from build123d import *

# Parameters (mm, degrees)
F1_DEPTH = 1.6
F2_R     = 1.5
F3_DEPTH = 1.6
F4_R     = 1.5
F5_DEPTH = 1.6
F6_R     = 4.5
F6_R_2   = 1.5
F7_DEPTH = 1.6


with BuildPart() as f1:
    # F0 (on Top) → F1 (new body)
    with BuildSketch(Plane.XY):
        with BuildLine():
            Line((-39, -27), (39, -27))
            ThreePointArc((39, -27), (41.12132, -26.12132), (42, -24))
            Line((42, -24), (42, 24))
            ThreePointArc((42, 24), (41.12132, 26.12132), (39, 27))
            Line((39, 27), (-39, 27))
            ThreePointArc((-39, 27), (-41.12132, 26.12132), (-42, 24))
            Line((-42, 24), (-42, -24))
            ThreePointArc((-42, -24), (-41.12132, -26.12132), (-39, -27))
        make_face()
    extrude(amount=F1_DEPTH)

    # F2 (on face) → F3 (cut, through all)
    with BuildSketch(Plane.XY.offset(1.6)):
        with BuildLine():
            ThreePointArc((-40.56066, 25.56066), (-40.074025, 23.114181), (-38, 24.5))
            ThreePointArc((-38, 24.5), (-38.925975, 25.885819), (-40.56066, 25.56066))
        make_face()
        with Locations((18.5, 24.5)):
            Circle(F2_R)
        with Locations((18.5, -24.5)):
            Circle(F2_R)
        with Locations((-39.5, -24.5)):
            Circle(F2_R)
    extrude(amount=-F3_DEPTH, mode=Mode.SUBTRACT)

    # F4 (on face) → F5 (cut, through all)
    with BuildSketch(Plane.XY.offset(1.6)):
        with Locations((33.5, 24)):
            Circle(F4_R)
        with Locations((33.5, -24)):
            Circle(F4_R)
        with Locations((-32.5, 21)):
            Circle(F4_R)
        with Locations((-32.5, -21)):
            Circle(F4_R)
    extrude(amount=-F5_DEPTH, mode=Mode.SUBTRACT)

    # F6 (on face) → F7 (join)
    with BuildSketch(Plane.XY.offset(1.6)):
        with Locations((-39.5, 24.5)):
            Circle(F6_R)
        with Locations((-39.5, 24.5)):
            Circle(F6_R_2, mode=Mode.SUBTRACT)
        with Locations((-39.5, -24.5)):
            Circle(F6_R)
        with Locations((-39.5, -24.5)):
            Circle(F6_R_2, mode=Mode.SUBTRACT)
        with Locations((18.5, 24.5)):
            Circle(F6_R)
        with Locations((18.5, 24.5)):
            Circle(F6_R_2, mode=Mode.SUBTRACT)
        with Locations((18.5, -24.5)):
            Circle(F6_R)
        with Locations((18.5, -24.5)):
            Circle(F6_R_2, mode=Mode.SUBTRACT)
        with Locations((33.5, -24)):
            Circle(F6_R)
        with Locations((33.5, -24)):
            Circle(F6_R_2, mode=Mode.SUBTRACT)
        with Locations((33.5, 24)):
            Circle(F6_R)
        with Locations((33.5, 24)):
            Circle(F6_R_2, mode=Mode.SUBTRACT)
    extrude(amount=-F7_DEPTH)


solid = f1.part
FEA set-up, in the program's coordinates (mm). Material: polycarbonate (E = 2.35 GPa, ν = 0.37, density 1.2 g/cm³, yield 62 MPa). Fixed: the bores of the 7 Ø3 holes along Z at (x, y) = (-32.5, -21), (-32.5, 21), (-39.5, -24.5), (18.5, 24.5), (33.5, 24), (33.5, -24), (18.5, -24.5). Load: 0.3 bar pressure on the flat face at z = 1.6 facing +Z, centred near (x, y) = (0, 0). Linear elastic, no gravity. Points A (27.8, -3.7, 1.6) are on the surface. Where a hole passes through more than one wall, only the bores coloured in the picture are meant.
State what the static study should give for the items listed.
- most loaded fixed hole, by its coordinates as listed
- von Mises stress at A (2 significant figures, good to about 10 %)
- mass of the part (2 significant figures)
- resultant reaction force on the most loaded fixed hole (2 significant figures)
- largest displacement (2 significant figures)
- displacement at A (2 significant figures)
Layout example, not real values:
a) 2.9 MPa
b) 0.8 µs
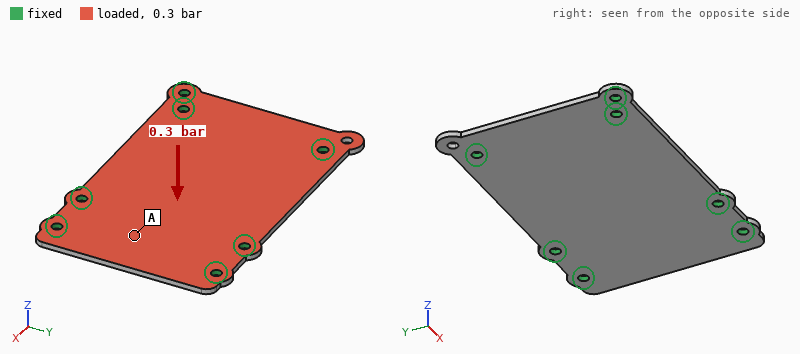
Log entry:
a) (-32.5, -21)
b) 6.6 MPa
c) 8.7 g
d) 33 N
e) 1.2 mm
f) 0.52 mm
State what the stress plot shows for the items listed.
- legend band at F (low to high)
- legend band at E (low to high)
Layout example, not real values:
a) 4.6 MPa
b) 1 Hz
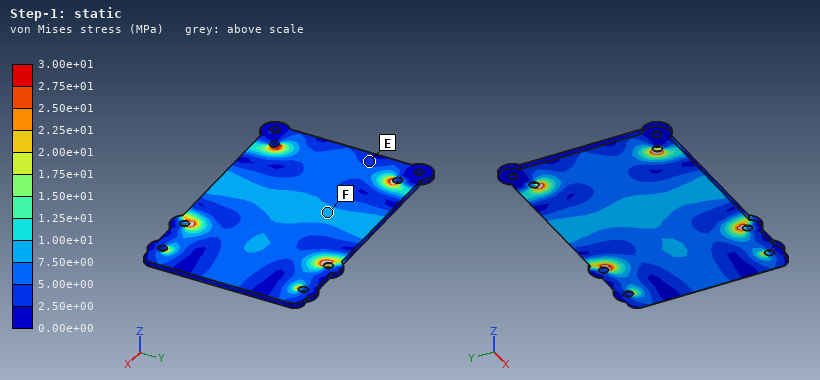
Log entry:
a) 7.50e+00 to 1.00e+01 MPa
b) 2.50e+00 to 5.00e+00 MPa
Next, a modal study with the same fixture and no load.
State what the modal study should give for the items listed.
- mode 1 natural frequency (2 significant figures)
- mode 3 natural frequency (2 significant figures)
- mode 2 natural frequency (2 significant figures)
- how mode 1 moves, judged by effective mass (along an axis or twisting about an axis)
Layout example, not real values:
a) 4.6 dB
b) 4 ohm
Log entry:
a) 700 Hz
b) 1100 Hz
c) 1100 Hz
d) along Z
